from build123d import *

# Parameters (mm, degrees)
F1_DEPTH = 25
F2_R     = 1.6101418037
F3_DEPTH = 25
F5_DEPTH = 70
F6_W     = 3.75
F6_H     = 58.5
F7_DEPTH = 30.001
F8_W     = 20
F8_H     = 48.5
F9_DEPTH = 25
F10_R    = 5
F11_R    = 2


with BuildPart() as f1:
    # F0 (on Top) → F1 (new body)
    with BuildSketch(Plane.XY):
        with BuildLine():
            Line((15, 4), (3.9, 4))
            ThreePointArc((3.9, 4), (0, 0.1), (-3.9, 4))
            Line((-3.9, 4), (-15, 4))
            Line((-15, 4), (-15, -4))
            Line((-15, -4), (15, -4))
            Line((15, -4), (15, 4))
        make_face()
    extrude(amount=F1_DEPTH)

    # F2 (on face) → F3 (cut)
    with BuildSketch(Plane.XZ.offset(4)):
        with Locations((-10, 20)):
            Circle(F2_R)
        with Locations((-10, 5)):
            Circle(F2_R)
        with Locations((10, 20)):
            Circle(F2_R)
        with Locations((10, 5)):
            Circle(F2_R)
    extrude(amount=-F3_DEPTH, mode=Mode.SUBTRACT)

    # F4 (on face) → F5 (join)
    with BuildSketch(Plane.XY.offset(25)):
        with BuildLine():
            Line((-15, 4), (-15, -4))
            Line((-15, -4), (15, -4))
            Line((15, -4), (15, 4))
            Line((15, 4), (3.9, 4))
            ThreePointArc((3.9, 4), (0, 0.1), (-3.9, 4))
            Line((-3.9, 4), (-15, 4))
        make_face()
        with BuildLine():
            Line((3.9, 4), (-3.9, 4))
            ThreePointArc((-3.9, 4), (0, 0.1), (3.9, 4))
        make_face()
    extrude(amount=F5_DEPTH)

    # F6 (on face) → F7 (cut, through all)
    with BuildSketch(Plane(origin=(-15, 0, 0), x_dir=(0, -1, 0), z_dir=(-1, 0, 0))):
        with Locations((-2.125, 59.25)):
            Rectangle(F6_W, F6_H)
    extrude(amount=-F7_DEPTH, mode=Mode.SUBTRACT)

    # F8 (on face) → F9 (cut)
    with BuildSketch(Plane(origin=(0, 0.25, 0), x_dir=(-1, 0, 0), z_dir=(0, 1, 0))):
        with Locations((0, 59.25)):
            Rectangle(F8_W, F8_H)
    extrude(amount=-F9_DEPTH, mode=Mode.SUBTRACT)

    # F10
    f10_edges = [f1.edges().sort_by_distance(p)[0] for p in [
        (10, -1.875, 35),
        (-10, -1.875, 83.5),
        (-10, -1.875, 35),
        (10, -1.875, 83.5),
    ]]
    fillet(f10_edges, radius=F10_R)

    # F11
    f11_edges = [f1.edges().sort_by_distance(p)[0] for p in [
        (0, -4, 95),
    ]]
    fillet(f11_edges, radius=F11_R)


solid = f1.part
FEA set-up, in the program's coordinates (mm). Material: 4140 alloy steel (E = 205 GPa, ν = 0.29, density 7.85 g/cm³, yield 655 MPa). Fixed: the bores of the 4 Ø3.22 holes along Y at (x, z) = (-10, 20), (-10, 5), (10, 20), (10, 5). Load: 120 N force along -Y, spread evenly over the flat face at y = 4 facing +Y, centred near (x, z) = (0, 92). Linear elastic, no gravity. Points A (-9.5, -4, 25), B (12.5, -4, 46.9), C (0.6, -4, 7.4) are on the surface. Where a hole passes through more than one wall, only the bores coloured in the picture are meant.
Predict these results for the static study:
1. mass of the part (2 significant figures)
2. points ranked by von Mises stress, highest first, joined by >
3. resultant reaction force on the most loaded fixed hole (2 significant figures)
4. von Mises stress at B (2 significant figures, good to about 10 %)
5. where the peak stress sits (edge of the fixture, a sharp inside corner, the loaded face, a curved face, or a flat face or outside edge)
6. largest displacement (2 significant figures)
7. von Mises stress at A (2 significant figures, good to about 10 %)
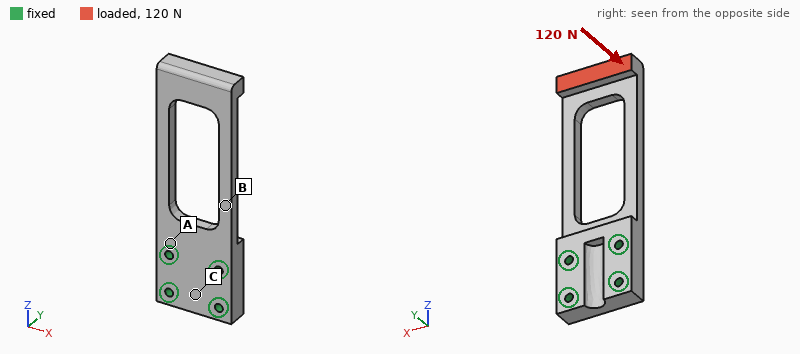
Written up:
89 g
B > A > C
130 N
180 MPa
a curved face
0.74 mm
38 MPa
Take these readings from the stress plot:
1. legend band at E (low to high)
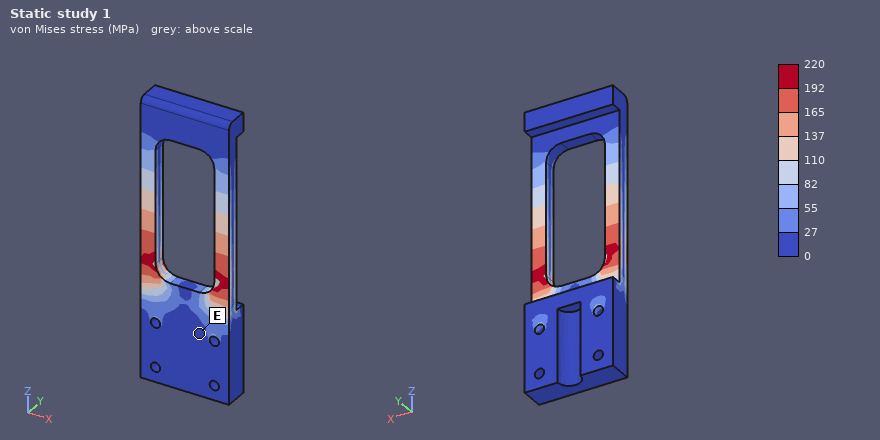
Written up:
0 to 27 MPa
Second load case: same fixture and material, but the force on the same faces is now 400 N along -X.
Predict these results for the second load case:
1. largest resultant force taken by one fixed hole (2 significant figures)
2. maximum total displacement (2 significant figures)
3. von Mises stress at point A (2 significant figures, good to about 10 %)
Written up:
1.2 kN
0.32 mm
38 MPa
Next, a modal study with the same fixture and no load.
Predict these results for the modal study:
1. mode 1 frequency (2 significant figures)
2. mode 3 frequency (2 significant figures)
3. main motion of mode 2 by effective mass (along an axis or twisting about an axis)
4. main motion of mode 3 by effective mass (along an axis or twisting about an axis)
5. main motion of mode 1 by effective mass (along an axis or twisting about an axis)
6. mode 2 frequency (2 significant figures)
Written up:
490 Hz
1900 Hz
along X
twisting about Z
along Y
1300 Hz
